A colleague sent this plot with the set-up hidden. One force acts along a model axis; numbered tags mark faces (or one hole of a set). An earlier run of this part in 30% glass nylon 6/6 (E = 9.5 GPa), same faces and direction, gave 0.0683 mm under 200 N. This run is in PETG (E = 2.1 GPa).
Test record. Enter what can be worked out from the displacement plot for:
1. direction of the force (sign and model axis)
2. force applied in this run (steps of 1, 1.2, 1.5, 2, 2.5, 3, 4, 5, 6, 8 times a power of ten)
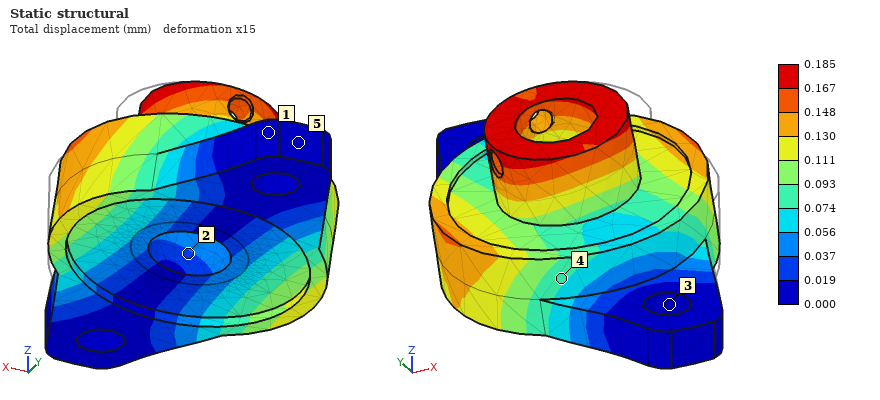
-X
120 N
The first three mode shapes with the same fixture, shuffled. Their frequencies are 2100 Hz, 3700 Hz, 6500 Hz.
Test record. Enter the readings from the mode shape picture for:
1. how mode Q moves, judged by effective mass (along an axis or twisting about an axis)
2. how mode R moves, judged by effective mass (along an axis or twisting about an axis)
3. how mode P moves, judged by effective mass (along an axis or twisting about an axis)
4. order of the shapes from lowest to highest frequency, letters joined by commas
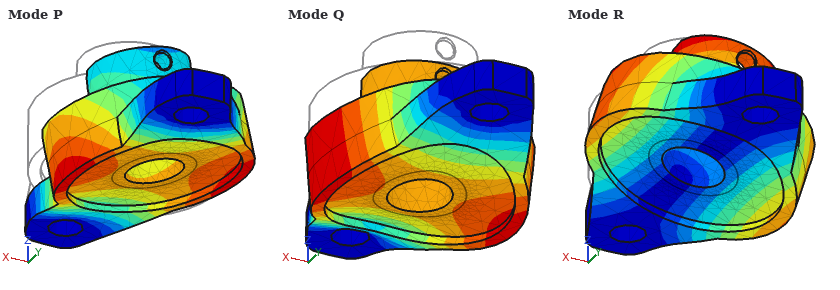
along Z
along X
along X
R, Q, P
